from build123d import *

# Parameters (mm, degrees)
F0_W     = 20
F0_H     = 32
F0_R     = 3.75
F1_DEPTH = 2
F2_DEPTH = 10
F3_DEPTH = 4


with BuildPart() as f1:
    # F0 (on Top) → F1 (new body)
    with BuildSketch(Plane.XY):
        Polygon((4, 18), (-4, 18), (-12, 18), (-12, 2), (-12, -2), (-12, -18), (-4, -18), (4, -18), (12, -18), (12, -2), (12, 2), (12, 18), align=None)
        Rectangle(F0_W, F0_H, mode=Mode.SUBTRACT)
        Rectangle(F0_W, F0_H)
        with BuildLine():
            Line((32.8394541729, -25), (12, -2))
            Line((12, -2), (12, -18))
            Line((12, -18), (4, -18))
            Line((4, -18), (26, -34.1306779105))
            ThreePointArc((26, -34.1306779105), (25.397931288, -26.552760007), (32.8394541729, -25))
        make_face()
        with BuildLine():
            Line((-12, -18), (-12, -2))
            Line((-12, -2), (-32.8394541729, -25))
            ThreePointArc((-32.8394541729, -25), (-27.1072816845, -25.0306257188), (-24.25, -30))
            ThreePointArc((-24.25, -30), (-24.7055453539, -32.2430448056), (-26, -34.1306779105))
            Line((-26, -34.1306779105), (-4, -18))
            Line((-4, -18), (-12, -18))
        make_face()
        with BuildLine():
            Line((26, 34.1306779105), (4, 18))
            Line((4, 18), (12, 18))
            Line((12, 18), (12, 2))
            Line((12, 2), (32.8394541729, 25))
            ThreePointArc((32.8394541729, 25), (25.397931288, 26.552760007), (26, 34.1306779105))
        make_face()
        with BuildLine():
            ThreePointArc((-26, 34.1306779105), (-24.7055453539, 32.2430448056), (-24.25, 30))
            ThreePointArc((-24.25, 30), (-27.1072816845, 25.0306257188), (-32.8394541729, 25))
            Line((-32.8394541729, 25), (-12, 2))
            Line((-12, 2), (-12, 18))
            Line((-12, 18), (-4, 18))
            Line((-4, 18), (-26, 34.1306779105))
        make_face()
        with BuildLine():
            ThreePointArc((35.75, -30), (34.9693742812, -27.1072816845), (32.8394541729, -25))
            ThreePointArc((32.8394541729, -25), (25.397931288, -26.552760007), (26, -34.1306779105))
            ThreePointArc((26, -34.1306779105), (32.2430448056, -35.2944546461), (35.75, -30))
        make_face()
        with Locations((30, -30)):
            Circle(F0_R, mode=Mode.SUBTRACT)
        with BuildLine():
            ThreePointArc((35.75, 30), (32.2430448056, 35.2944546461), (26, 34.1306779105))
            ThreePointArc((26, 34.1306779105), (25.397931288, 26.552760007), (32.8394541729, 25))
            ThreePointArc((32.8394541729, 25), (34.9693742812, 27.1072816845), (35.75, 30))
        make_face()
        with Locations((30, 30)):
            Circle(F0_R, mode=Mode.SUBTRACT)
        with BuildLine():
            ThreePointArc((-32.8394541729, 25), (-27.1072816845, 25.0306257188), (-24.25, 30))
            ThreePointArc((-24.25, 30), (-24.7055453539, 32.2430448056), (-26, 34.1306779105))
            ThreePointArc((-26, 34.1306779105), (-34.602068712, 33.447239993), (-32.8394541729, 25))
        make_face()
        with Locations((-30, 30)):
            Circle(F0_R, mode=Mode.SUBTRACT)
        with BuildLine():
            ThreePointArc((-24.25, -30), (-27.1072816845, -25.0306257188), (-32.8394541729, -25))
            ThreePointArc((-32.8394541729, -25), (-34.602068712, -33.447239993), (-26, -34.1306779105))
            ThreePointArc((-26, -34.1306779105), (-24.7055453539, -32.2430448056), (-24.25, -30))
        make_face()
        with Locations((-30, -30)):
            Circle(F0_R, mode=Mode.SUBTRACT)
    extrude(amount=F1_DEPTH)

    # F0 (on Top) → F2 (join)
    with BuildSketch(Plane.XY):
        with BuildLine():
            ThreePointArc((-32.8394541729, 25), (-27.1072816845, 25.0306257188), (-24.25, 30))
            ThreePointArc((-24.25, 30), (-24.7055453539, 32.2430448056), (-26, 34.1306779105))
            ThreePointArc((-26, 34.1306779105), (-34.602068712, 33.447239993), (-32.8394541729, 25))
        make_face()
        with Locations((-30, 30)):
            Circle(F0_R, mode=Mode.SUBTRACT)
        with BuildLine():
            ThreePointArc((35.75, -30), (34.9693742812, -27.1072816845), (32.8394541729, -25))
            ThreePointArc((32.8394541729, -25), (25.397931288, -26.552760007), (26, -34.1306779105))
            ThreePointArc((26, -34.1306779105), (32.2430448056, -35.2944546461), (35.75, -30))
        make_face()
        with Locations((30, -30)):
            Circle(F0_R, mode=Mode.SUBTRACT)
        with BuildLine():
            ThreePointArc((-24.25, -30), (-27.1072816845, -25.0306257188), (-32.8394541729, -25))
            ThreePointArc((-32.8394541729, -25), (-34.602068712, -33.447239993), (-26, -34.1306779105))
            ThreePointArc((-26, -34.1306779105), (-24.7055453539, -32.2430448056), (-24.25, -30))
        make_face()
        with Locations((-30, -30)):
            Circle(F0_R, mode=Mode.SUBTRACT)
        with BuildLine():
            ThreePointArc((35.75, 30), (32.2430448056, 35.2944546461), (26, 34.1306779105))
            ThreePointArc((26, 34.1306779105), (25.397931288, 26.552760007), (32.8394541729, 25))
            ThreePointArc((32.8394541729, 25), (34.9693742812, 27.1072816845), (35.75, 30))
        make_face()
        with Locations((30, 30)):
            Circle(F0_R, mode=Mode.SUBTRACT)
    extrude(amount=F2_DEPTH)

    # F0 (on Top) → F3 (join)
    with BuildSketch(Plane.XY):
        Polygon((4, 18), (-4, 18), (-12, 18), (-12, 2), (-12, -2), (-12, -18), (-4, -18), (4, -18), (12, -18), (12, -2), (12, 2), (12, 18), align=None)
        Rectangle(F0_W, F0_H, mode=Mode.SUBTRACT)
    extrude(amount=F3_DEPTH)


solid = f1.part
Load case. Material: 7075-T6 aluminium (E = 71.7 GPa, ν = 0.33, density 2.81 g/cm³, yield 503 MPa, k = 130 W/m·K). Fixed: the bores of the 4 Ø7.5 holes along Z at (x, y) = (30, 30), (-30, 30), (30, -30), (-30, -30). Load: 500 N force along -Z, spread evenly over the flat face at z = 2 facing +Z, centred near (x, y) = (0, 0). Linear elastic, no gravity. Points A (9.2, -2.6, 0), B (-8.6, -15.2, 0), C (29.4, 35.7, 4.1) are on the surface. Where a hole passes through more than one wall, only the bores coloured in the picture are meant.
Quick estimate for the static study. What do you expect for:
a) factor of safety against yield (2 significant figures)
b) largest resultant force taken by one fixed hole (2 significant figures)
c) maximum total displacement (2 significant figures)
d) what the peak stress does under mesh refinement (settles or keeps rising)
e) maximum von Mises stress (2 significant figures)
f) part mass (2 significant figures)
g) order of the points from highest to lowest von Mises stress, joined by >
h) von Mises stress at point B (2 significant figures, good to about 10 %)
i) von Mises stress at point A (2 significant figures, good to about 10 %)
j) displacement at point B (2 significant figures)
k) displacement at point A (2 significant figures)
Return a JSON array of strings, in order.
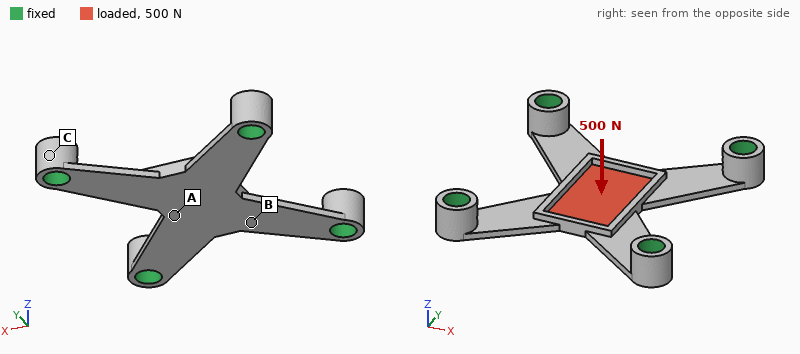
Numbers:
["2.9", "170 N", "0.33 mm", "settles", "170 MPa", "20 g", "A > B > C", "47 MPa", "69 MPa", "0.23 mm", "0.30 mm"]
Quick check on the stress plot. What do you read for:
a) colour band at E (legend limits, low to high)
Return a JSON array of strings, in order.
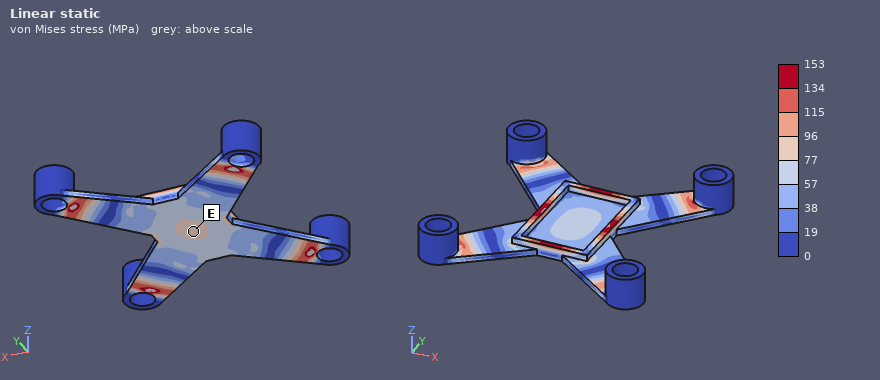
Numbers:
["77 to 96 MPa"]
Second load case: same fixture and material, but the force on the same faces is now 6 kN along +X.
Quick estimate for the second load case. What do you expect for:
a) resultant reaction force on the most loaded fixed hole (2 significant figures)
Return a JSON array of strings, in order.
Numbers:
["1.9 kN"]
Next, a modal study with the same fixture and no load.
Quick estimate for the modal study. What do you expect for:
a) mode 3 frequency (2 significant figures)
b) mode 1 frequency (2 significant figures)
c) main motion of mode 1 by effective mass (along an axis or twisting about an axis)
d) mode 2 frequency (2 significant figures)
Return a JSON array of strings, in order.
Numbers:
["5500 Hz", "2500 Hz", "along Z", "5000 Hz"]
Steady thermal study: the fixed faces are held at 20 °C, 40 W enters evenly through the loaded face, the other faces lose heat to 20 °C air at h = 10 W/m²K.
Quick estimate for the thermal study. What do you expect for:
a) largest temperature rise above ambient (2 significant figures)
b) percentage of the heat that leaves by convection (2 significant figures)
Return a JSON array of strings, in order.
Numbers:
["76 K", "5.0 %"]
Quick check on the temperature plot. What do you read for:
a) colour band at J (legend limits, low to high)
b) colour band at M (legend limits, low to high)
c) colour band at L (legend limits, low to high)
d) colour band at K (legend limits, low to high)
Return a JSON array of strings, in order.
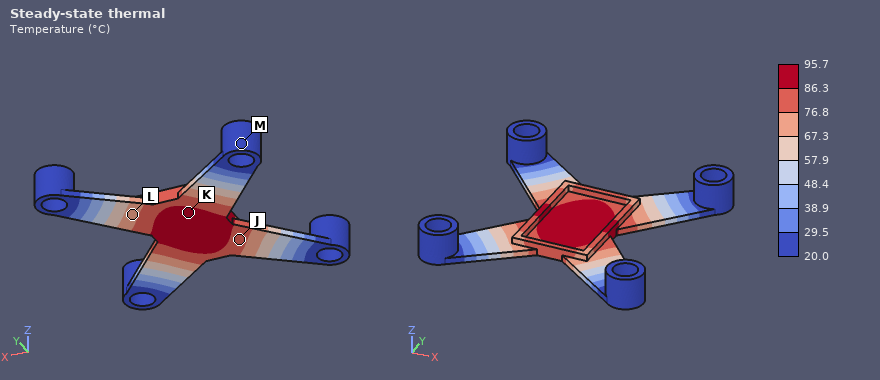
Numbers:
["76.8 to 86.3 °C", "20.0 to 29.5 °C", "67.3 to 76.8 °C", "86.3 to 95.7 °C"]
